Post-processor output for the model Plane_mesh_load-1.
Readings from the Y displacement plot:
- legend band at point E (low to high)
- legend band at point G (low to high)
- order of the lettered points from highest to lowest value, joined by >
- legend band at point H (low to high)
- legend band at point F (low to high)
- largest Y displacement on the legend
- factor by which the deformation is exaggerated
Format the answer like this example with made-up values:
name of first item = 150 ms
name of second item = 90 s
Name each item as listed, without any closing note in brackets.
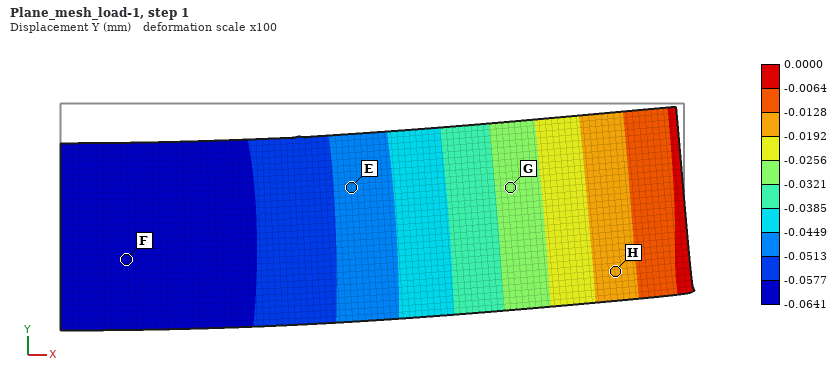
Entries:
legend band at point E = -0.0513 to -0.0449 mm
legend band at point G = -0.0321 to -0.0256 mm
order of the lettered points from highest to lowest value, joined by > = H > G > E > F
legend band at point H = -0.0192 to -0.0128 mm
legend band at point F = -0.0641 to -0.0577 mm
largest Y displacement on the legend = 0.0000 mm
factor by which the deformation is exaggerated = 100
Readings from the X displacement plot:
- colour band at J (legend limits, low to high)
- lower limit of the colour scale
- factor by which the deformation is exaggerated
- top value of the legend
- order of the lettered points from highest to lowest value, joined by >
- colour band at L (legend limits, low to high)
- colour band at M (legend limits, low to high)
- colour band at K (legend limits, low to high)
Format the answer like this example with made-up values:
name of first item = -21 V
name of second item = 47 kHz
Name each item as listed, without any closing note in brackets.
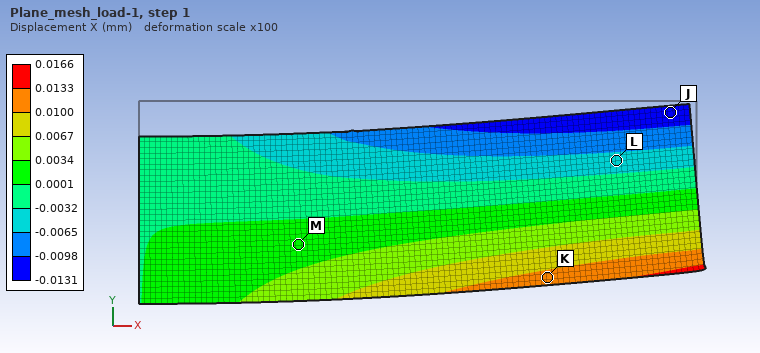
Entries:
colour band at J = -0.0131 to -0.0098 mm
lower limit of the colour scale = -0.0131 mm
factor by which the deformation is exaggerated = 100
top value of the legend = 0.0166 mm
order of the lettered points from highest to lowest value, joined by > = K > M > L > J
colour band at L = -0.0065 to -0.0032 mm
colour band at M = 0.0001 to 0.0034 mm
colour band at K = 0.0100 to 0.0133 mm
